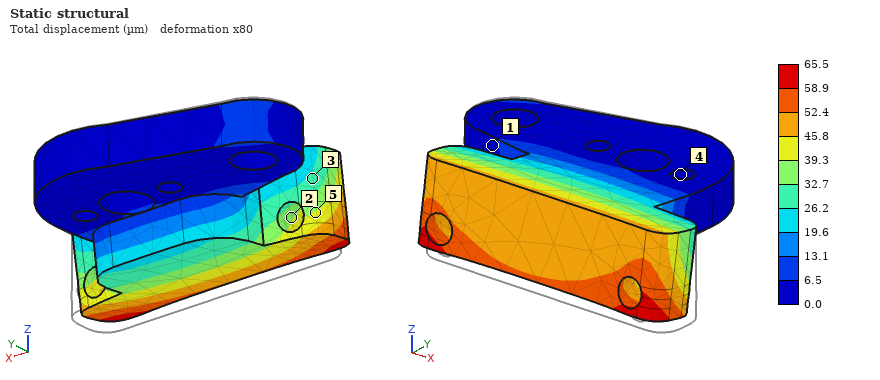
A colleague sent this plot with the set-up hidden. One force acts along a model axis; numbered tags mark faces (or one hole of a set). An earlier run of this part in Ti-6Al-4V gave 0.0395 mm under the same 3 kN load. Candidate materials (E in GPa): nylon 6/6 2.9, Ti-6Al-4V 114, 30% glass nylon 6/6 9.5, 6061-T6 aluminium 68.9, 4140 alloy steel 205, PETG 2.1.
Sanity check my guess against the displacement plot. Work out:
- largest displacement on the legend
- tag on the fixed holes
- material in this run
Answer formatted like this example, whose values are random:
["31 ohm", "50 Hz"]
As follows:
["65.5 µm", "4", "6061-T6 aluminium"]
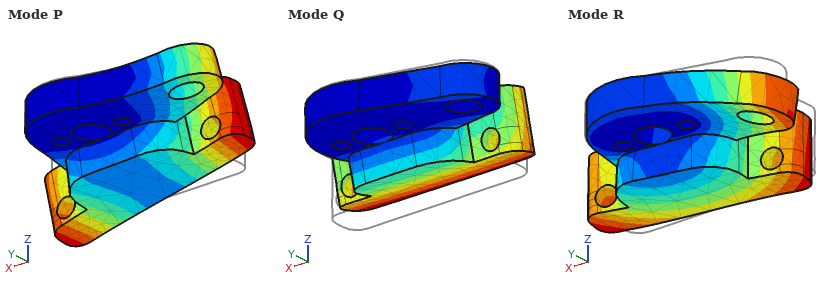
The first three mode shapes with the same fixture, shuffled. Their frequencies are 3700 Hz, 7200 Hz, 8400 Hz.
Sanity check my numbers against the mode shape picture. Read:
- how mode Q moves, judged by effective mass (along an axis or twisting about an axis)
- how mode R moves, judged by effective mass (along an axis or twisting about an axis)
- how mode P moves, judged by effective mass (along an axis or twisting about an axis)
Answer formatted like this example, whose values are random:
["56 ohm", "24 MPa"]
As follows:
["along Z", "along X", "twisting about Y"]
